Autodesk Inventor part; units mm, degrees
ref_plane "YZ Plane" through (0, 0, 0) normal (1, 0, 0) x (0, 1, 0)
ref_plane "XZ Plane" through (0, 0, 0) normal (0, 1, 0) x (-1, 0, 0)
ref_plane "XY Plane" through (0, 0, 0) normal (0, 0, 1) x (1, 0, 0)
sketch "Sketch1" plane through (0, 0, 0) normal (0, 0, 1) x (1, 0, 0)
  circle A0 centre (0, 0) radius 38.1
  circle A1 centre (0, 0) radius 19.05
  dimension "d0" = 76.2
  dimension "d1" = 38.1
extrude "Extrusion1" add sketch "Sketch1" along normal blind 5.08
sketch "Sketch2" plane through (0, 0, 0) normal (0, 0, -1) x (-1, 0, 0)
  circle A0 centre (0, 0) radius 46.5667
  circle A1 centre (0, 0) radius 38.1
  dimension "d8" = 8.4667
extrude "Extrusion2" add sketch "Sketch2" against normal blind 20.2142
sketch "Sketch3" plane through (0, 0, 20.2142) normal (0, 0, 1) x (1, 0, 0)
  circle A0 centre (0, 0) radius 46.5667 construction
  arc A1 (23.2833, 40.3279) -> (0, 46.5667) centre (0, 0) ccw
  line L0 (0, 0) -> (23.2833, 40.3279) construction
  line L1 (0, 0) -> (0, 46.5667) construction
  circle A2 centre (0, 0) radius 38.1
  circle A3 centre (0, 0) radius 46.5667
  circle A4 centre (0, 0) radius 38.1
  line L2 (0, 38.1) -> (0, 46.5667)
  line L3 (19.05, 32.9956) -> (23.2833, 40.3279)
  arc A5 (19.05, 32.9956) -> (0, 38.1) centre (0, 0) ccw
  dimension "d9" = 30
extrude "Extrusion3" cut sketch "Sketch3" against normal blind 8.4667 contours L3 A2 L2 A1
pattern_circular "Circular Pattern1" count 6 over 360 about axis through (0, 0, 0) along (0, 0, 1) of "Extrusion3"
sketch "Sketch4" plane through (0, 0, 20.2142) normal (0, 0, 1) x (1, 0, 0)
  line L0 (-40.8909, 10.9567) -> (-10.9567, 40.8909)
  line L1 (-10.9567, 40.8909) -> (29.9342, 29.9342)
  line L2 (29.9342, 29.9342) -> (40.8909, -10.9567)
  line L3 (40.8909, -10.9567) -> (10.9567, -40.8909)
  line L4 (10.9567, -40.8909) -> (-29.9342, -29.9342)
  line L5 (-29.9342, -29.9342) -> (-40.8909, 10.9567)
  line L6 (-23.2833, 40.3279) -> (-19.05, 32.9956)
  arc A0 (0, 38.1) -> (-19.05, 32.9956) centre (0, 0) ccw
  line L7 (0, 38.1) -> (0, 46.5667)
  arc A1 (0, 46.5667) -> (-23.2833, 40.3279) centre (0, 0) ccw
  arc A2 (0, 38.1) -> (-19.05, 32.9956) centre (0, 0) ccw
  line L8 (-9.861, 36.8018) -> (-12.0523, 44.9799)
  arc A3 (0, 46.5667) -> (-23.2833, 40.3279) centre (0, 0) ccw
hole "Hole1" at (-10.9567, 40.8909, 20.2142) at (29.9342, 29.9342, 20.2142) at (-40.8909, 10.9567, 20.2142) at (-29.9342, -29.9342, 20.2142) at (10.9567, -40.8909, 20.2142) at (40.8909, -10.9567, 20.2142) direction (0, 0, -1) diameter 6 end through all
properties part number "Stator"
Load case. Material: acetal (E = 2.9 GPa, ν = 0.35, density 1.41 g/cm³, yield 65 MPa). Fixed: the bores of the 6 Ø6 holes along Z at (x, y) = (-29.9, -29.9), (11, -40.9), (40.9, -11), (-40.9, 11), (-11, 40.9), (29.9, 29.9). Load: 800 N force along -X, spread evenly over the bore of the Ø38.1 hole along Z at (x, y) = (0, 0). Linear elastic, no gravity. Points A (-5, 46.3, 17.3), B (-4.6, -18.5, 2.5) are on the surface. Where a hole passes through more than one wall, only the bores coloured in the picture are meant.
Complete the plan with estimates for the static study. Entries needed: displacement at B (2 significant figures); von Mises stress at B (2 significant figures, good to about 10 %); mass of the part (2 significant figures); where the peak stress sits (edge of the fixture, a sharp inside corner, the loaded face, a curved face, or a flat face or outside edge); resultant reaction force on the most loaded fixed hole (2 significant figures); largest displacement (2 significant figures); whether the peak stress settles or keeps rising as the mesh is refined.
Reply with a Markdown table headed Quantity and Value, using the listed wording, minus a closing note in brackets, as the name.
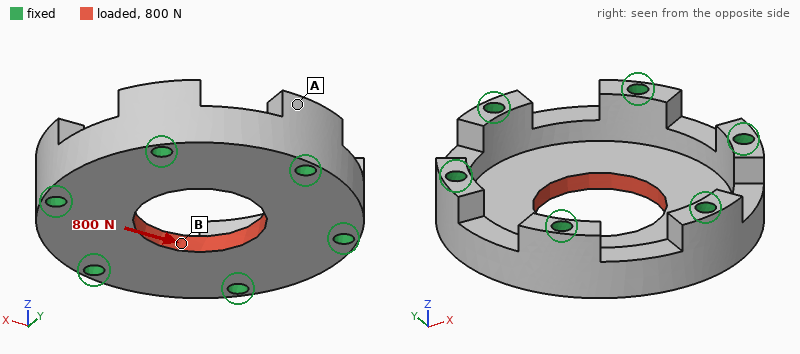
| Quantity | Value |
|---|---|
| displacement at B | 14 µm |
| von Mises stress at B | 2.2 MPa |
| mass of the part | 70 g |
| where the peak stress sits | edge of the fixture |
| resultant reaction force on the most loaded fixed hole | 180 N |
| largest displacement | 17 µm |
| whether the peak stress settles or keeps rising as the mesh is refined | keeps rising |
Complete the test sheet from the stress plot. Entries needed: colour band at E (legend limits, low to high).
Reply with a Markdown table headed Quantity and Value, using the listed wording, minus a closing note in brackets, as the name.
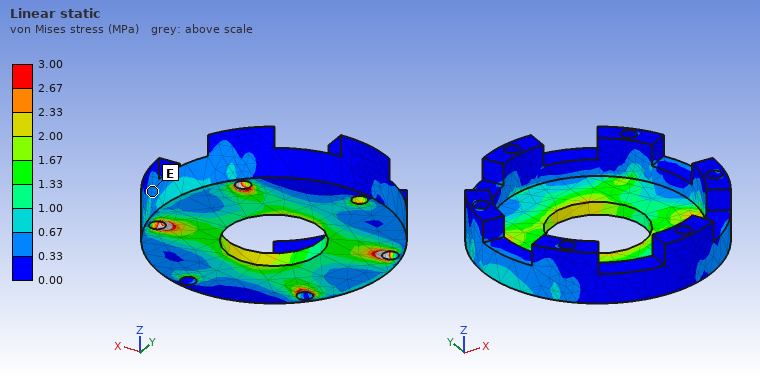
| Quantity | Value |
|---|---|
| colour band at E | 0.33 to 0.67 MPa |
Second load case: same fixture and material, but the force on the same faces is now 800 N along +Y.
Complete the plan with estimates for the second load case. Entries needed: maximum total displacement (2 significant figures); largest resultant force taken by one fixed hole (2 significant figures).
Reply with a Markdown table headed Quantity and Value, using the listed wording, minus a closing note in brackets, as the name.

| Quantity | Value |
|---|---|
| maximum total displacement | 17 µm |
| largest resultant force taken by one fixed hole | 180 N |
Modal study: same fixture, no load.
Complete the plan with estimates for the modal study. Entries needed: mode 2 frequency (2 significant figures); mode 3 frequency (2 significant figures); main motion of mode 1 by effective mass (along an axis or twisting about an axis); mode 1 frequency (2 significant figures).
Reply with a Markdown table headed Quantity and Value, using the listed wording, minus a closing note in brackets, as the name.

| Quantity | Value |
|---|---|
| mode 2 frequency | 3800 Hz |
| mode 3 frequency | 3800 Hz |
| main motion of mode 1 by effective mass | along Z |
| mode 1 frequency | 3100 Hz |
